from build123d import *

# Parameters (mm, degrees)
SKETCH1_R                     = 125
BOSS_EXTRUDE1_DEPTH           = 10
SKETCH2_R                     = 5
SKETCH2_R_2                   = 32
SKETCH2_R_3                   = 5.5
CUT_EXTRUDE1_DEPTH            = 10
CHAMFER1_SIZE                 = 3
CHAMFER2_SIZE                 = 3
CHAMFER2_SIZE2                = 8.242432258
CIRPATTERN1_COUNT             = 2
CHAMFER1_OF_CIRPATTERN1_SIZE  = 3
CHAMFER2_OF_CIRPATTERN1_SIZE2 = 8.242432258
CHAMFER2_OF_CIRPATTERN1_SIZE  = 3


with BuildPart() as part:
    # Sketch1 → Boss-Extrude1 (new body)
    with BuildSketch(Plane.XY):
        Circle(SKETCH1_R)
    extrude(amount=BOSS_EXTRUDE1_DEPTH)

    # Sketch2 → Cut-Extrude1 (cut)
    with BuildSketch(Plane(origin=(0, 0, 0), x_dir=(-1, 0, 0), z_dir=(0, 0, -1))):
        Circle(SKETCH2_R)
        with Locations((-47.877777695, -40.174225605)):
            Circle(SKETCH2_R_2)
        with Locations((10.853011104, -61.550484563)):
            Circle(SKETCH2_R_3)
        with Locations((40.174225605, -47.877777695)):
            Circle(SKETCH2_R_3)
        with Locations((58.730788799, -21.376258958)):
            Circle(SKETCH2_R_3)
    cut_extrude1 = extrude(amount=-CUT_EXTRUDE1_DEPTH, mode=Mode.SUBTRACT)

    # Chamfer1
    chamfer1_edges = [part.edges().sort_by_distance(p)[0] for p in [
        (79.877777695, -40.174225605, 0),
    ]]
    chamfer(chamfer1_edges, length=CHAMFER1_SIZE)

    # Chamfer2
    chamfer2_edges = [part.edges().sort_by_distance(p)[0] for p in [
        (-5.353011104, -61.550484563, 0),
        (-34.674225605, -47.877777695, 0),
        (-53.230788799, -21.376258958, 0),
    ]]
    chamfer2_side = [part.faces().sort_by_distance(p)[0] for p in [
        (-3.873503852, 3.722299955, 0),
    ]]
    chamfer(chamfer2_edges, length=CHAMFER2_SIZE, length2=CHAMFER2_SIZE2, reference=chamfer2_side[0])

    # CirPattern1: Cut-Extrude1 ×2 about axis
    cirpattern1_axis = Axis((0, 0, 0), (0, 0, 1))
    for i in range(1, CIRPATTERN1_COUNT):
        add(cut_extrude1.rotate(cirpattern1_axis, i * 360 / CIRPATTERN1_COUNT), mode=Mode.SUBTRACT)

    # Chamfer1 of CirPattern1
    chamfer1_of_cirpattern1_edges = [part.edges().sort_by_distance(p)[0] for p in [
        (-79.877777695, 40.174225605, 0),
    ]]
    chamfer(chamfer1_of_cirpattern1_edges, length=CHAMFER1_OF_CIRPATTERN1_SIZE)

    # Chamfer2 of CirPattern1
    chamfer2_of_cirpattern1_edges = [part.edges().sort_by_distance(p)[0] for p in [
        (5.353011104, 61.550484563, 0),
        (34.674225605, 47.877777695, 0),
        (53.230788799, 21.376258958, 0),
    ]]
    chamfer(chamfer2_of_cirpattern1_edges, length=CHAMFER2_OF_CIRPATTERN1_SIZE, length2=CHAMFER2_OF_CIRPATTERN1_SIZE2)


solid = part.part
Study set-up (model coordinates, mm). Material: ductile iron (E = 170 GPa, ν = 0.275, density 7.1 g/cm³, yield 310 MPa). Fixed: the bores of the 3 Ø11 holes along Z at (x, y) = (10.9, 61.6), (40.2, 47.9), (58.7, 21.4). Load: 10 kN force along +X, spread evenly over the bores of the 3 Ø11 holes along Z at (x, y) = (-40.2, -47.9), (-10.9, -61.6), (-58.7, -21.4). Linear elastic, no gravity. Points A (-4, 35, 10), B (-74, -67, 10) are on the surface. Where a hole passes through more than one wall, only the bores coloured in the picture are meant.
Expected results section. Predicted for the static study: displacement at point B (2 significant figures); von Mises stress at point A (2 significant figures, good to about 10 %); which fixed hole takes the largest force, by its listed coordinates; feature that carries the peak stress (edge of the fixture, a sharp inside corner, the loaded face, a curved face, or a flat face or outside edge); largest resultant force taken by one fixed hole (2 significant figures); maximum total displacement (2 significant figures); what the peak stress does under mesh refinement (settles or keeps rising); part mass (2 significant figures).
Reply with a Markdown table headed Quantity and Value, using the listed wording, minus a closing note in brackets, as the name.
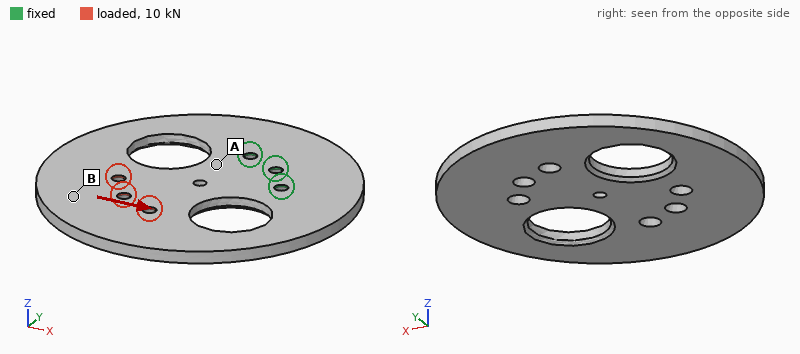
| Quantity | Value |
|---|---|
| displacement at point B | 0.18 mm |
| von Mises stress at point A | 22 MPa |
| which fixed hole takes the largest force, by its listed coordinates | (58.7, 21.4) |
| feature that carries the peak stress | edge of the fixture |
| largest resultant force taken by one fixed hole | 15 kN |
| maximum total displacement | 0.25 mm |
| what the peak stress does under mesh refinement | keeps rising |
| part mass | 2.9 kg |
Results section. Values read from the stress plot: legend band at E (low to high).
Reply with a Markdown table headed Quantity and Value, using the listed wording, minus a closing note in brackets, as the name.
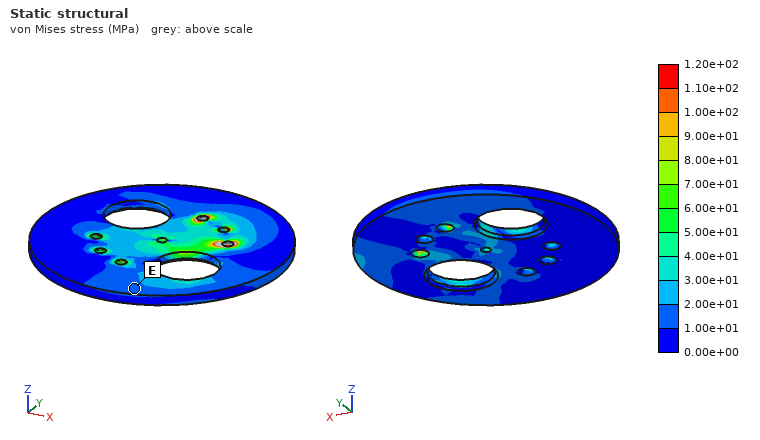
| Quantity | Value |
|---|---|
| legend band at E | 1.00e+01 to 2.00e+01 MPa |
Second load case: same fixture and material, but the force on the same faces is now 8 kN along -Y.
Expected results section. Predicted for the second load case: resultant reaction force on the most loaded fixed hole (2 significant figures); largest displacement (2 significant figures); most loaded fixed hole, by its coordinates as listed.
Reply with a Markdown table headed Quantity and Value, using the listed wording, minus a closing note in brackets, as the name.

| Quantity | Value |
|---|---|
| resultant reaction force on the most loaded fixed hole | 11 kN |
| largest displacement | 0.21 mm |
| most loaded fixed hole, by its coordinates as listed | (10.9, 61.6) |
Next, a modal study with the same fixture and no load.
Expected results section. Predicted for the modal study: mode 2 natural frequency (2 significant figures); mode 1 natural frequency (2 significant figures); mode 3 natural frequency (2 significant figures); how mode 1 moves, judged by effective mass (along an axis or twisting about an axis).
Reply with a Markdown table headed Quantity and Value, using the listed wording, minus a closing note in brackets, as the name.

| Quantity | Value |
|---|---|
| mode 2 natural frequency | 430 Hz |
| mode 1 natural frequency | 190 Hz |
| mode 3 natural frequency | 800 Hz |
| how mode 1 moves, judged by effective mass | along Z |
